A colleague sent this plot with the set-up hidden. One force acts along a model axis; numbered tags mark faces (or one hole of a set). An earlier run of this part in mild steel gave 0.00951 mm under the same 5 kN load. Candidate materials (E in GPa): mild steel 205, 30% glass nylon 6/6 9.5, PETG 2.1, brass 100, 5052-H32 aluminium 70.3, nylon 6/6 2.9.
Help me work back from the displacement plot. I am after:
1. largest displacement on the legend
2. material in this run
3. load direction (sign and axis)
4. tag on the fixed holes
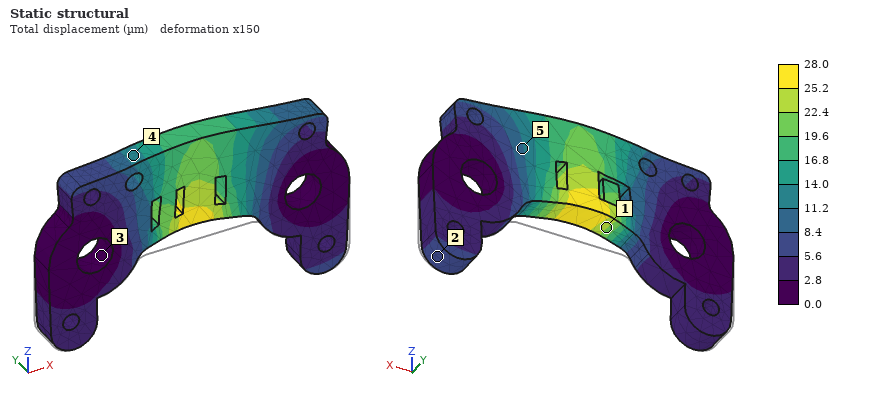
28.0 µm
5052-H32 aluminium
+Z
3
